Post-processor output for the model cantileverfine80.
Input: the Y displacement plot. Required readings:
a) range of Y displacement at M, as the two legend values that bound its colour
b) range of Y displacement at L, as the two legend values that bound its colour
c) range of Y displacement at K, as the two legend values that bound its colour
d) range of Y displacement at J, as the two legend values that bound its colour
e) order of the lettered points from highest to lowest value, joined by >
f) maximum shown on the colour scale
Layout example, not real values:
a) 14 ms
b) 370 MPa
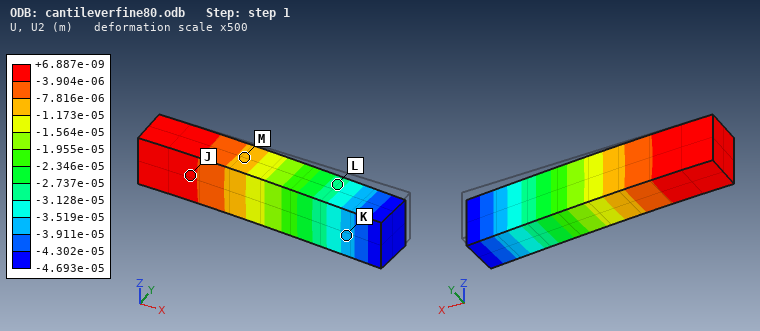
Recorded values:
a) -1.173e-05 to -7.816e-06 m
b) -3.128e-05 to -2.737e-05 m
c) -3.911e-05 to -3.519e-05 m
d) -3.904e-06 to +6.887e-09 m
e) J > M > L > K
f) +6.887e-09 m
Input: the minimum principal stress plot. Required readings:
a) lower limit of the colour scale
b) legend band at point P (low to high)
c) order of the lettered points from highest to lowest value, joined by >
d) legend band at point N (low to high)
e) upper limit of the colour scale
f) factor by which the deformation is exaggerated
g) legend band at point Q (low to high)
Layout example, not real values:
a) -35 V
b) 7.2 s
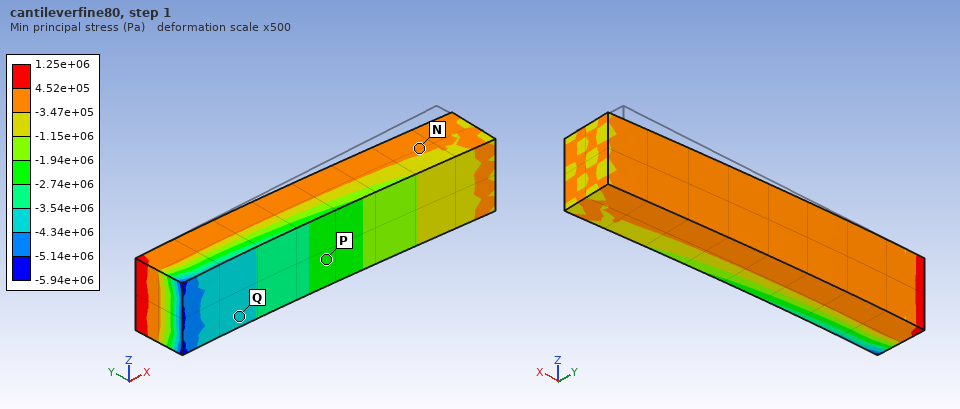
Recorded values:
a) -5.94e+06 Pa
b) -2.74e+06 to -1.94e+06 Pa
c) N > P > Q
d) -3.47e+05 to 4.52e+05 Pa
e) 1.25e+06 Pa
f) 500
g) -4.34e+06 to -3.54e+06 Pa
